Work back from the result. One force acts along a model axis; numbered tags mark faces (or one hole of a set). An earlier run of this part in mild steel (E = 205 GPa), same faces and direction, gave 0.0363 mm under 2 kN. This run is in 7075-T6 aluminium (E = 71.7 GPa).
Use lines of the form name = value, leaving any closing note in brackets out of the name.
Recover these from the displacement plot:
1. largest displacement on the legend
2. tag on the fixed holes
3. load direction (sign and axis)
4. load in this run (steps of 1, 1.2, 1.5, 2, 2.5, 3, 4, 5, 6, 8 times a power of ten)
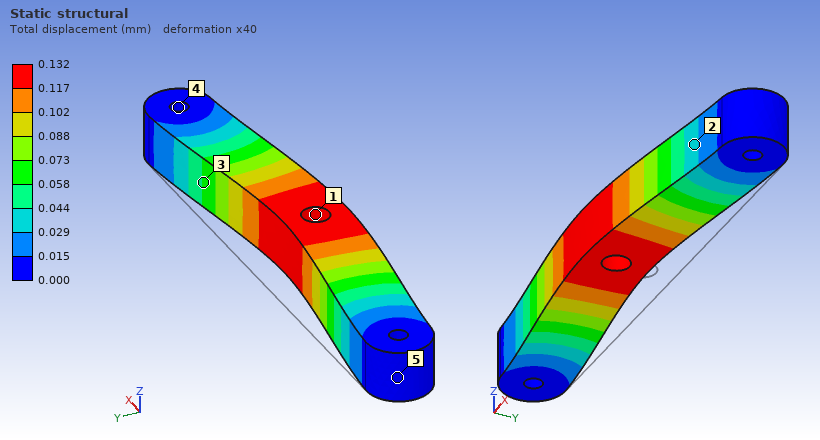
largest displacement on the legend = 0.132 mm
tag on the fixed holes = 4
load direction = -Y
load in this run = 2.5 kN
